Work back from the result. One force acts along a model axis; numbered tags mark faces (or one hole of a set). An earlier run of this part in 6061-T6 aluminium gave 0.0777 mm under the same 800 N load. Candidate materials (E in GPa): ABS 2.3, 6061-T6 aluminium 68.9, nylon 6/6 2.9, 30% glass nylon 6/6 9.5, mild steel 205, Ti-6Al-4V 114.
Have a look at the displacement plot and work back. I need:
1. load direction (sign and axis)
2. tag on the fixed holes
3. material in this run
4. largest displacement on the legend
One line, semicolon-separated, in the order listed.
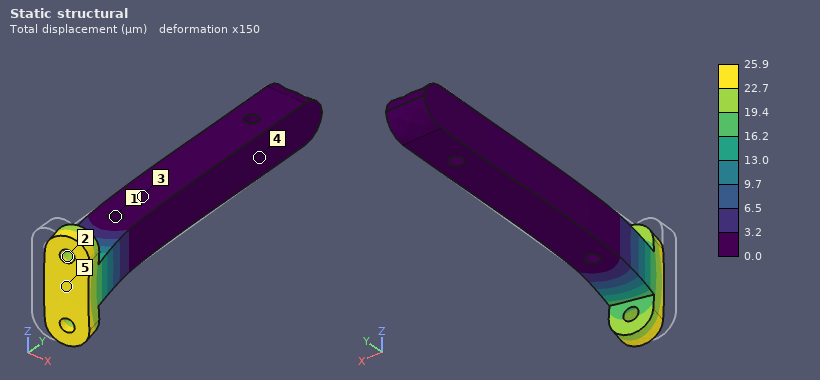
+X; 1; mild steel; 25.9 µm
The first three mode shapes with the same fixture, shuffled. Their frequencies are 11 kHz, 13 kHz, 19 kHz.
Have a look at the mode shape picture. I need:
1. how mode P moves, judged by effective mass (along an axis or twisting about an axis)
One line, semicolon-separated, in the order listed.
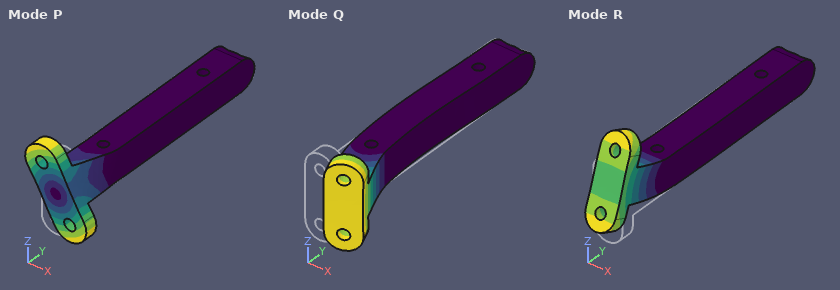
twisting about Y
